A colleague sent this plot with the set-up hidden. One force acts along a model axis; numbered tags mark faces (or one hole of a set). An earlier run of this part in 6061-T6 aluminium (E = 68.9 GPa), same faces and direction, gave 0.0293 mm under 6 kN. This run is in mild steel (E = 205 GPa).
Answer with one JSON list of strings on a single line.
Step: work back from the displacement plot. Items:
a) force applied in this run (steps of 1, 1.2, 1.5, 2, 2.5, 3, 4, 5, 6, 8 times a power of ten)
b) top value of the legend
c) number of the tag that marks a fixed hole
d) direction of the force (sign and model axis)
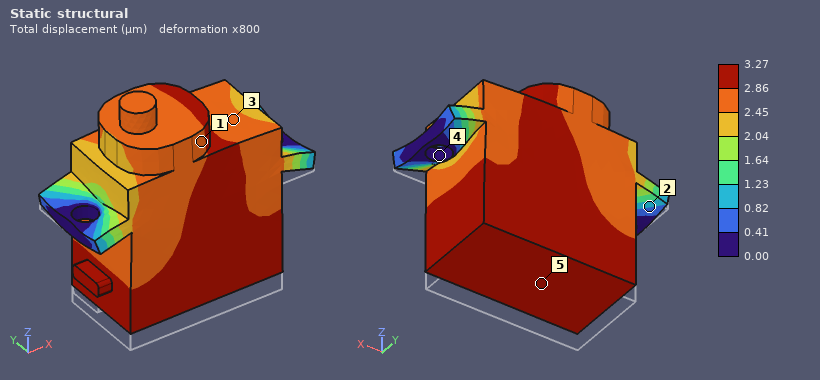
["2 kN", "3.27 µm", "4", "+Z"]
